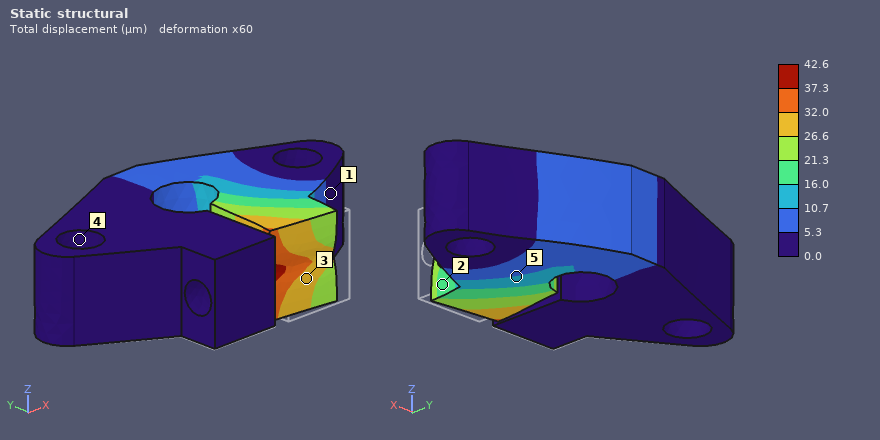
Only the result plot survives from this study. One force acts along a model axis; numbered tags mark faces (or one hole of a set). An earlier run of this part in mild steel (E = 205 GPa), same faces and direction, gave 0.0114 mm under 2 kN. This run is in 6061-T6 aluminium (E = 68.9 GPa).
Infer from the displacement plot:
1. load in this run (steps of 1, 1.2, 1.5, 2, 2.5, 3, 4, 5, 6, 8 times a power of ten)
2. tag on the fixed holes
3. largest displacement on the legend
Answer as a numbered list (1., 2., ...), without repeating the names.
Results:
1. 2.5 kN
2. 4
3. 42.6 µm
